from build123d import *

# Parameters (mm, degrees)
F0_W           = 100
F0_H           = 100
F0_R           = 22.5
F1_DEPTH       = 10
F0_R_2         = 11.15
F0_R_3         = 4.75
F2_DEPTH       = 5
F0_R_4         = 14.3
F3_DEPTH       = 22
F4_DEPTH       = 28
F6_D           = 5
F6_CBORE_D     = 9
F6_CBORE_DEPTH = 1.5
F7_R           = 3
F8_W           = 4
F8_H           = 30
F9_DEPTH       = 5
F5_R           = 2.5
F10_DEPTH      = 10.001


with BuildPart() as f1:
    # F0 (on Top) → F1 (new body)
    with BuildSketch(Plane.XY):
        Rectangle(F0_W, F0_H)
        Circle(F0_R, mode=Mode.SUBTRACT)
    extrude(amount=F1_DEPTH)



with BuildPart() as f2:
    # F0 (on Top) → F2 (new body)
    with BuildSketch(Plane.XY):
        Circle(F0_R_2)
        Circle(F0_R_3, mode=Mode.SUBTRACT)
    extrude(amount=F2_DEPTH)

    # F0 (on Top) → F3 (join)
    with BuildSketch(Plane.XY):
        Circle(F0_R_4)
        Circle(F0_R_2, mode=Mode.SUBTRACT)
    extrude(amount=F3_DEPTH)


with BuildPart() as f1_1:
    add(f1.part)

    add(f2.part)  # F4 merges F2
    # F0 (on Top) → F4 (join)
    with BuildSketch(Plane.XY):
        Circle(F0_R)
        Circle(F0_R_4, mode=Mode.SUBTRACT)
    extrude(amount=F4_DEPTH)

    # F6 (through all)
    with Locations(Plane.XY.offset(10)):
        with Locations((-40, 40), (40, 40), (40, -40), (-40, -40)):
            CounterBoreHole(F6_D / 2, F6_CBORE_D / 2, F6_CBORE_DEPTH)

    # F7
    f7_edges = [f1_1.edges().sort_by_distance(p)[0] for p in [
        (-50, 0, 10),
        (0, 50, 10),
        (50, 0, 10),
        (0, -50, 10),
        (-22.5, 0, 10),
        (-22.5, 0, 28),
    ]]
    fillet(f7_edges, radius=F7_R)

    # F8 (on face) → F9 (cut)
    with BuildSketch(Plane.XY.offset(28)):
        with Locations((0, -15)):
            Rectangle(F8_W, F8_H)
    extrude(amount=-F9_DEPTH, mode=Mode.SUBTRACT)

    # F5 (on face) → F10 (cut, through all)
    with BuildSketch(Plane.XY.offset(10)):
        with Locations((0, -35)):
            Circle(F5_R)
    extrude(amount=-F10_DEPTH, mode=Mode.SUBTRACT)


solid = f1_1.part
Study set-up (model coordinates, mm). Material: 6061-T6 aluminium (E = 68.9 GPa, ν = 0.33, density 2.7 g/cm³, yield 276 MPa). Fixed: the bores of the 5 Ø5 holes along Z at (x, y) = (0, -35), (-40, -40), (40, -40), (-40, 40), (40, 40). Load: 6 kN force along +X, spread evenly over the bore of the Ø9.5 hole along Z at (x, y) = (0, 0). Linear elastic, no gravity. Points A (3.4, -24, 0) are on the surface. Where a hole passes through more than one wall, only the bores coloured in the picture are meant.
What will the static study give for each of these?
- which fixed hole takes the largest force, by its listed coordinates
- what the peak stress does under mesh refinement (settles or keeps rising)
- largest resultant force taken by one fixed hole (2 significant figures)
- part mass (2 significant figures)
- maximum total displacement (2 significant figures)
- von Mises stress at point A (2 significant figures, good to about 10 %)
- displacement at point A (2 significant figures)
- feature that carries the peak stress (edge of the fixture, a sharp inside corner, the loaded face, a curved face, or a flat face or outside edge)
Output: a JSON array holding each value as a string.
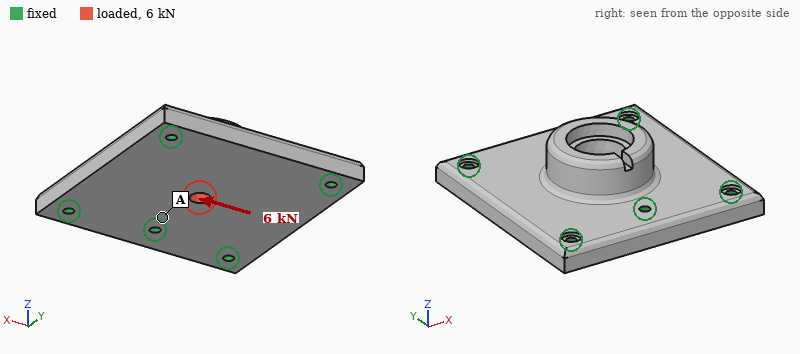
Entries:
["(0, -35)", "keeps rising", "1.7 kN", "310 g", "11 µm", "7.3 MPa", "2.6 µm", "a sharp inside corner"]
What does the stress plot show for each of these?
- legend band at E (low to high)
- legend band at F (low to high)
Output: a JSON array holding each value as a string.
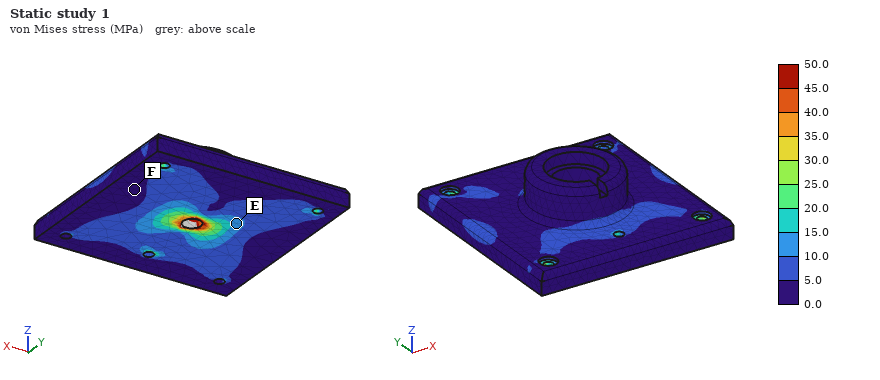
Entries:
["10.0 to 15.0 MPa", "0.0 to 5.0 MPa"]
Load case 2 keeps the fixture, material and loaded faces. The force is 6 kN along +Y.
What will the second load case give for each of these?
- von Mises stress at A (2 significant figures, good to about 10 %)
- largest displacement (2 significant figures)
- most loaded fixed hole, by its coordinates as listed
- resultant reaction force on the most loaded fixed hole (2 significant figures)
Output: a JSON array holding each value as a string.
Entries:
["14 MPa", "10 µm", "(0, -35)", "2.3 kN"]
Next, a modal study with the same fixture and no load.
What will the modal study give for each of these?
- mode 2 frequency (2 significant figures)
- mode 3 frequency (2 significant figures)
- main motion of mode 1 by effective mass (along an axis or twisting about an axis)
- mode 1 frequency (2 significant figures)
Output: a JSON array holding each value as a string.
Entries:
["6900 Hz", "8500 Hz", "along Z", "5200 Hz"]
